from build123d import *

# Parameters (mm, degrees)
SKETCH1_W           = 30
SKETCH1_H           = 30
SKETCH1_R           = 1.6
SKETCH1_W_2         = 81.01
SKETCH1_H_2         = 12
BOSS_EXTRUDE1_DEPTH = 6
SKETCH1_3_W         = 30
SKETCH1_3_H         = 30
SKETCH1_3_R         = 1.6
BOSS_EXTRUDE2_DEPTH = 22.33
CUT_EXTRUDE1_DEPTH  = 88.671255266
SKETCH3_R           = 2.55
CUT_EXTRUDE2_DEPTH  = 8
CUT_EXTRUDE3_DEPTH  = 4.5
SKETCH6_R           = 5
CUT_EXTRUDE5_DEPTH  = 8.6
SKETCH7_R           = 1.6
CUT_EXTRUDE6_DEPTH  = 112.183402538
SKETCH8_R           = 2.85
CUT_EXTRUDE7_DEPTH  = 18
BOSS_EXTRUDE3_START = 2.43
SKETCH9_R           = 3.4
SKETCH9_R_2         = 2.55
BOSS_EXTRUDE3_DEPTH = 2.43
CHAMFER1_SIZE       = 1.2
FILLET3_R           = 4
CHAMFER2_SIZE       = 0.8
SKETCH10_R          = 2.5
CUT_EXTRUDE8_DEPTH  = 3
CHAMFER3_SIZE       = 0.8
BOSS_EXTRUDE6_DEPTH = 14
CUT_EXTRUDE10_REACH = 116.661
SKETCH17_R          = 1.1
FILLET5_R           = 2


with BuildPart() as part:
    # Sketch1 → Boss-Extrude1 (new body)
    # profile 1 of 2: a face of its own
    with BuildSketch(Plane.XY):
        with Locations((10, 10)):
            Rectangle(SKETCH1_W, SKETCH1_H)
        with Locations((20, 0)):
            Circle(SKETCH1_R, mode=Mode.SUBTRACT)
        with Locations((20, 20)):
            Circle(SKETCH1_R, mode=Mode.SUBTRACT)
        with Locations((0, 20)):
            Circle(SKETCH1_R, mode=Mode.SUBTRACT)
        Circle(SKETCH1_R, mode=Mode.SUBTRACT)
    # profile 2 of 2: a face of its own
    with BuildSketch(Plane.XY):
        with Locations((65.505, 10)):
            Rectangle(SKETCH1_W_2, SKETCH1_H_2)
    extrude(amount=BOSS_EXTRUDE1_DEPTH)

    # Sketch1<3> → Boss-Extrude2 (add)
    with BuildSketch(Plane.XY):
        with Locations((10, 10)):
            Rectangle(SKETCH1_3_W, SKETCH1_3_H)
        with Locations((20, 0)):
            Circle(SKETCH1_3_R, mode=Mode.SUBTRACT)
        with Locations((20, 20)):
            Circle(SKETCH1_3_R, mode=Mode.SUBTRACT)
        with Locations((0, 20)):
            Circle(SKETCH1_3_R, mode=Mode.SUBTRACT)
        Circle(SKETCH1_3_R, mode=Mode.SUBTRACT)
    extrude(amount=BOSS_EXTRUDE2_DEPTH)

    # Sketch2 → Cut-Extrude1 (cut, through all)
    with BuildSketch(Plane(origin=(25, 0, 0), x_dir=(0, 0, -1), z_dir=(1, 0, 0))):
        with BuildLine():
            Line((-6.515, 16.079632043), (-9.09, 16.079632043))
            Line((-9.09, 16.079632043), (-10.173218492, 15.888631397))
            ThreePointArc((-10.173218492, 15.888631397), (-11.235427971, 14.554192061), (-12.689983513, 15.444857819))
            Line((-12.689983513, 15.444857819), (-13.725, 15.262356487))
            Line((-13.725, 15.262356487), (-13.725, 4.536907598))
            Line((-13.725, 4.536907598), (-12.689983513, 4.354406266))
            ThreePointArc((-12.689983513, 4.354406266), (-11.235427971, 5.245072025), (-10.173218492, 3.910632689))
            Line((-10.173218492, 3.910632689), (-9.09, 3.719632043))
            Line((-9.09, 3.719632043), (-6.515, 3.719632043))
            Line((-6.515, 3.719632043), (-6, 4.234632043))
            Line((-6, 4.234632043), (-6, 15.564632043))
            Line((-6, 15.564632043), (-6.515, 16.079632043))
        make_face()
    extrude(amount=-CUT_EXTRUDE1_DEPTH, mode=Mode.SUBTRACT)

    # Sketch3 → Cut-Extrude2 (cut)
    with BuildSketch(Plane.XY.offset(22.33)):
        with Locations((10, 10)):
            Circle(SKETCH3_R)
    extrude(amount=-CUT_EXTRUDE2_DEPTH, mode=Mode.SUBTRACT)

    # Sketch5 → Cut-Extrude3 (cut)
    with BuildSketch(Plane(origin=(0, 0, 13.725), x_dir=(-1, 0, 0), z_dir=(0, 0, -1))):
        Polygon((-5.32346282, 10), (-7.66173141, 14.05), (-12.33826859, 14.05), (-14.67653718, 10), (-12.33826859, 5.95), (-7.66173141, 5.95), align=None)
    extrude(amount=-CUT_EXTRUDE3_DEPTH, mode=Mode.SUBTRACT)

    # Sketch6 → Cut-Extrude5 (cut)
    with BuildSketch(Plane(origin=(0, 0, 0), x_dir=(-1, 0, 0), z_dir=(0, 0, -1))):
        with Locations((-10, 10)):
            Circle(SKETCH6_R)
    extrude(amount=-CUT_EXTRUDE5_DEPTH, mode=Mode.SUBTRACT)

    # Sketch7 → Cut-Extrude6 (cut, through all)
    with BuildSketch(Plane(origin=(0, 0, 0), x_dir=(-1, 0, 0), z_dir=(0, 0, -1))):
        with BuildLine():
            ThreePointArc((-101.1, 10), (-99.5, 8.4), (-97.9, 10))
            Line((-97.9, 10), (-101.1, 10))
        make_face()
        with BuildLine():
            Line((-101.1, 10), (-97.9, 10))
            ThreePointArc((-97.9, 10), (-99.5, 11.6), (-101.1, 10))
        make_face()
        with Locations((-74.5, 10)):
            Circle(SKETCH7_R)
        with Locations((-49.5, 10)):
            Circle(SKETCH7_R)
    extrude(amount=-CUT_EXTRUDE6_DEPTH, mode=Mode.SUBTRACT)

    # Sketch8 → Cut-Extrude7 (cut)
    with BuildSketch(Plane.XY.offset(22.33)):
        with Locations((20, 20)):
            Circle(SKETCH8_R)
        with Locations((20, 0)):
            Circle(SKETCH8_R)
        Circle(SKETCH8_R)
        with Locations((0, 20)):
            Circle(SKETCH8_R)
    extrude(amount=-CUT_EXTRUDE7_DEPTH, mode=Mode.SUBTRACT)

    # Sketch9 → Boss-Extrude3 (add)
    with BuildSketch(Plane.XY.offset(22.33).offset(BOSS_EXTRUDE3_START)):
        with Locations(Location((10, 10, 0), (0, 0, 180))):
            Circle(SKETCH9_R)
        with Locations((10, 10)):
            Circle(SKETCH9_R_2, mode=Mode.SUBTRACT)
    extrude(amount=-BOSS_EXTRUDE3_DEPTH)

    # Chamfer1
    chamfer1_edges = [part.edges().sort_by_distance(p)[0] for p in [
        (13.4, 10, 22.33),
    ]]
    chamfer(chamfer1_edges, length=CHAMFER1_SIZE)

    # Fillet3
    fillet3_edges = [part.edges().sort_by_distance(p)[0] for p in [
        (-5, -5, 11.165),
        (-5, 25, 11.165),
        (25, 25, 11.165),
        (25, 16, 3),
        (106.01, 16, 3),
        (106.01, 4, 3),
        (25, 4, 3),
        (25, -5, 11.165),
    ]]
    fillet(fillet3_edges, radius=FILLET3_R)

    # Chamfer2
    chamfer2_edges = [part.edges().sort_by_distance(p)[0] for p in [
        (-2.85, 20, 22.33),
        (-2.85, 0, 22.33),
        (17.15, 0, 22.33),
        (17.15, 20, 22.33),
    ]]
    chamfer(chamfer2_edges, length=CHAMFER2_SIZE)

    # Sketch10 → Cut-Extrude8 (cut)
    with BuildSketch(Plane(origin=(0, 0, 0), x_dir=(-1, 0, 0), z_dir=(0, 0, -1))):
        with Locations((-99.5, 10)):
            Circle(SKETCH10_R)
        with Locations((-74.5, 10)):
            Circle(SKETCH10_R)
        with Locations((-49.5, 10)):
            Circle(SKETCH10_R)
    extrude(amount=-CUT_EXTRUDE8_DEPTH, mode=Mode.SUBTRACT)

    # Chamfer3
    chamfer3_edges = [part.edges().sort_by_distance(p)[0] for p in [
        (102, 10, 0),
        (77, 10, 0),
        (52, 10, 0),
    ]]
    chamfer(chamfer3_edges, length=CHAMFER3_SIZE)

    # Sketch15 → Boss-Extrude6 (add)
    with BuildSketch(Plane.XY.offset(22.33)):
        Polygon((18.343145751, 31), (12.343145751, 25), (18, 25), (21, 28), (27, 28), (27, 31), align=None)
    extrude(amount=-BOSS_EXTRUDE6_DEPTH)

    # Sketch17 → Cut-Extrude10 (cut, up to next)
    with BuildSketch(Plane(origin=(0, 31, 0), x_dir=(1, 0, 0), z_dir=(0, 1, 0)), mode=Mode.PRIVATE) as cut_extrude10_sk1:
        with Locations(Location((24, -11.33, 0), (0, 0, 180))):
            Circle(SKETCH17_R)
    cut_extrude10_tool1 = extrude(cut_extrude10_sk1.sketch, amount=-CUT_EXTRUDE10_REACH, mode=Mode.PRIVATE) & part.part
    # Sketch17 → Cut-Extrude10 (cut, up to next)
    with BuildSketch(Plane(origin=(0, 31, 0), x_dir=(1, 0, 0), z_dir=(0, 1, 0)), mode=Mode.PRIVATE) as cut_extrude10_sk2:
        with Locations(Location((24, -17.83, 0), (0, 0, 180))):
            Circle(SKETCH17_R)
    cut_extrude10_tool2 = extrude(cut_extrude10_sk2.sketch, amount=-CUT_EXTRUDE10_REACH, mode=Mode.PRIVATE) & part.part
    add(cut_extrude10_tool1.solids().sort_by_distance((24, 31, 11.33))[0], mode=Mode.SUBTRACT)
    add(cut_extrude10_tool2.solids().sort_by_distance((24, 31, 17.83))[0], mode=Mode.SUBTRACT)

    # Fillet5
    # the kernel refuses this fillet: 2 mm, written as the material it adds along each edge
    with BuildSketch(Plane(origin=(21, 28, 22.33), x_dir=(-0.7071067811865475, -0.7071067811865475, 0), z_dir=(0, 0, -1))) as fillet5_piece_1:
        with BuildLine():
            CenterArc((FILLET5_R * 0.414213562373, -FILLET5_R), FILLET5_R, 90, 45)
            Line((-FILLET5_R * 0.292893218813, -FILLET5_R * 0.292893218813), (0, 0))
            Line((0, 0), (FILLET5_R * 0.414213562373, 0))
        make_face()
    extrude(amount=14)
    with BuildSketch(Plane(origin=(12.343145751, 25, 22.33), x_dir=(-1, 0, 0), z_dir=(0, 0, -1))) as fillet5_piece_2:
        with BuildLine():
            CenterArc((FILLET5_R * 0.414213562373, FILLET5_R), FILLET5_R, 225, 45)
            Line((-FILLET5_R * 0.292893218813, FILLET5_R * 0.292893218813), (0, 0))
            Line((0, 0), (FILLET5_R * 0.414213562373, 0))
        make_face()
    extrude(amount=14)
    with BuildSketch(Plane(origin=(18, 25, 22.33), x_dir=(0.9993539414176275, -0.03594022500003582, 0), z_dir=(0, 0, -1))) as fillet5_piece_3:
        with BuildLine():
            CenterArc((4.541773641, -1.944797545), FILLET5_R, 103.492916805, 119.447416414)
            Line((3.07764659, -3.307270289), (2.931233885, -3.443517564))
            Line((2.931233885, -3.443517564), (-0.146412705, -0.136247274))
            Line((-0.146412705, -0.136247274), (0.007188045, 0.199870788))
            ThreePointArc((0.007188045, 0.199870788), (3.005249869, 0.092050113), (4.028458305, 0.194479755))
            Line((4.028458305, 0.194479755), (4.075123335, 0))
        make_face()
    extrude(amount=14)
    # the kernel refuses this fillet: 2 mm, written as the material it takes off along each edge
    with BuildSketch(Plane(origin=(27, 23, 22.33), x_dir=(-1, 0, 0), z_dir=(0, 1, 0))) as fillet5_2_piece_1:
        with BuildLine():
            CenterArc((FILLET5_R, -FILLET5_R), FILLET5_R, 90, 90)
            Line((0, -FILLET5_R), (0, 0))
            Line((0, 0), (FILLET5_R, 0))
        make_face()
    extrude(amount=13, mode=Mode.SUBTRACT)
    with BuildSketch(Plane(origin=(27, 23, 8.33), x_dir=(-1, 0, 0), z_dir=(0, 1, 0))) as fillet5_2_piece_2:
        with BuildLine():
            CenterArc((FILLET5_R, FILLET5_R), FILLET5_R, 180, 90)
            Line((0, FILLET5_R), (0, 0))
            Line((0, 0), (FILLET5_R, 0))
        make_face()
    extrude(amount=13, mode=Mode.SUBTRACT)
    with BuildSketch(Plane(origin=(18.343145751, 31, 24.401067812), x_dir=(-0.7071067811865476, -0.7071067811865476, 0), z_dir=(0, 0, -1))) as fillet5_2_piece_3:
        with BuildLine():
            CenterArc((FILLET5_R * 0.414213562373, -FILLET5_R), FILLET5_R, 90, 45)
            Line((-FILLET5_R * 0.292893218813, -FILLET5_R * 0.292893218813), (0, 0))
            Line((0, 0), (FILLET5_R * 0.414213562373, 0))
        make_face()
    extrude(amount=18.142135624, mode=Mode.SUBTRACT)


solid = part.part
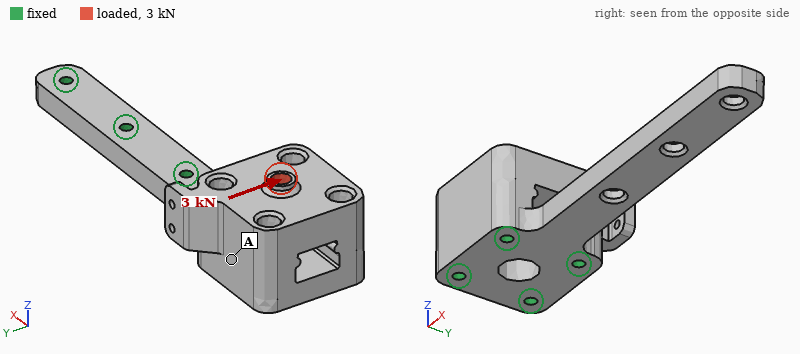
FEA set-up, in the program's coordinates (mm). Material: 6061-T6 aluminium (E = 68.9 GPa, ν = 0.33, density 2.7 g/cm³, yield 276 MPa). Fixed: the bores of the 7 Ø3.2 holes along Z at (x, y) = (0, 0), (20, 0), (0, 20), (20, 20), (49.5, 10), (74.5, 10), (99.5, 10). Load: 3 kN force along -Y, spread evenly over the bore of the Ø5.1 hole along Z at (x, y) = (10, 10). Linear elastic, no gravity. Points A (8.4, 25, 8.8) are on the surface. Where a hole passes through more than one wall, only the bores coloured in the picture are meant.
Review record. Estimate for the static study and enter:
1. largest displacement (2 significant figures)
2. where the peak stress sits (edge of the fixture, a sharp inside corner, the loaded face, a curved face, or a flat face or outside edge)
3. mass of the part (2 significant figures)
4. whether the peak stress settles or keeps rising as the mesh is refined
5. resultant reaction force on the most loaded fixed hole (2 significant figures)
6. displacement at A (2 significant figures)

30 µm
edge of the fixture
56 g
keeps rising
1.4 kN
12 µm
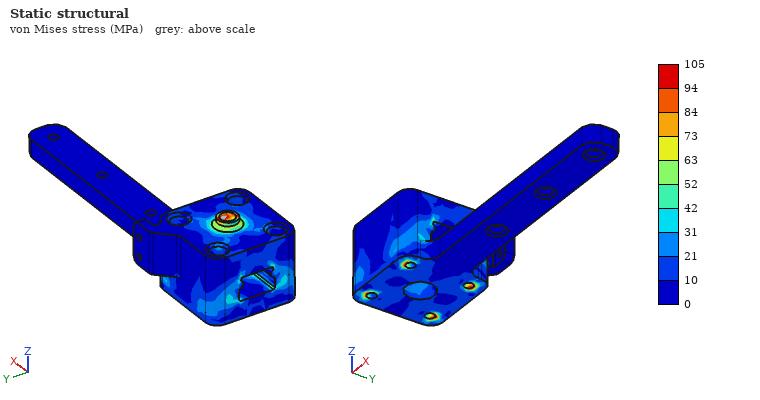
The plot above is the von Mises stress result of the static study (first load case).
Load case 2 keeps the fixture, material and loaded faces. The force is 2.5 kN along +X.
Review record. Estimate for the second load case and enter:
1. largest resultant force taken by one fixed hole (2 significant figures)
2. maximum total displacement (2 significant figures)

1.3 kN
21 µm
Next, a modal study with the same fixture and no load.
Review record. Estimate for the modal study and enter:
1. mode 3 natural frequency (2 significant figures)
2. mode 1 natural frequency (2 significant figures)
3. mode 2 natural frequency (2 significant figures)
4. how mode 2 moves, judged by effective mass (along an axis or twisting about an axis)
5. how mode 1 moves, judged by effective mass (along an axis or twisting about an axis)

23 kHz
14 kHz
18 kHz
along X
along Y
